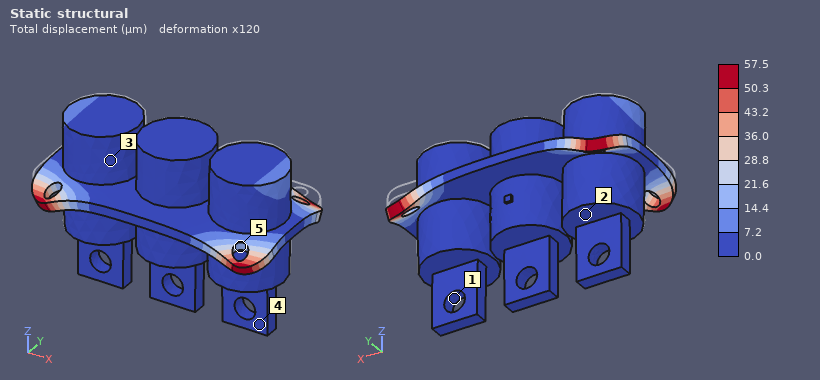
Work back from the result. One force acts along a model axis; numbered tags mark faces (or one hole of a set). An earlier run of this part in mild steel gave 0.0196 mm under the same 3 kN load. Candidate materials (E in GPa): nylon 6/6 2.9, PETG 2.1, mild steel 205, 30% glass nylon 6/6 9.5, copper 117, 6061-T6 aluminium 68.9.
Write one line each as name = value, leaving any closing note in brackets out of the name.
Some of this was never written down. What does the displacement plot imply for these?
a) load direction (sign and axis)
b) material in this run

load direction = -Z
material in this run = 6061-T6 aluminium
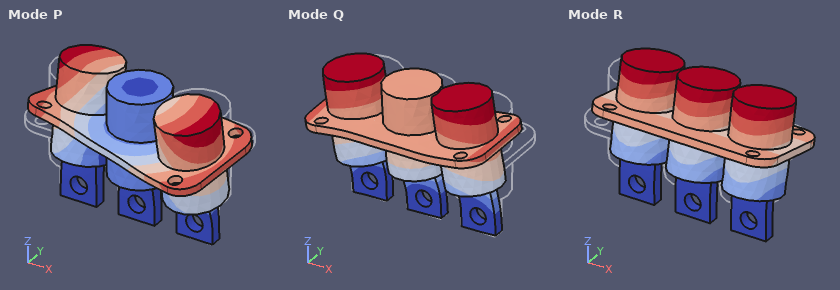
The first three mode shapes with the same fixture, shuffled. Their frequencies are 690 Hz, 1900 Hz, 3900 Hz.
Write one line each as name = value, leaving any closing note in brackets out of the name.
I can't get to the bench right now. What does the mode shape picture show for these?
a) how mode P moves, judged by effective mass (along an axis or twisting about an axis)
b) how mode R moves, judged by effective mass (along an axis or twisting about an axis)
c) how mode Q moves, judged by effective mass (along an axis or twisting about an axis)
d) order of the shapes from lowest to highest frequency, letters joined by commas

how mode P moves, judged by effective mass = twisting about Z
how mode R moves, judged by effective mass = along Y
how mode Q moves, judged by effective mass = along X
order of the shapes from lowest to highest frequency, letters joined by commas = R, P, Q
